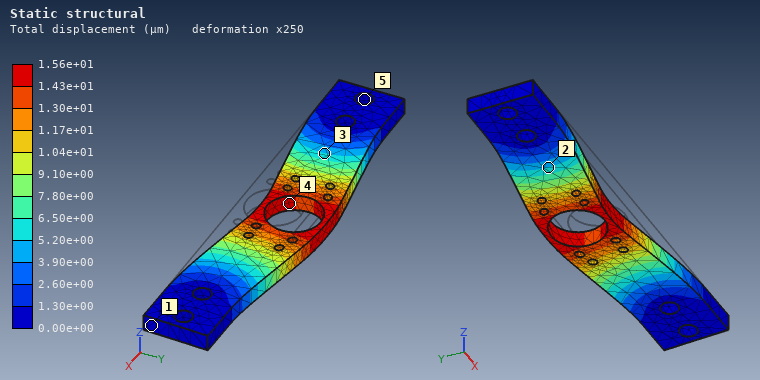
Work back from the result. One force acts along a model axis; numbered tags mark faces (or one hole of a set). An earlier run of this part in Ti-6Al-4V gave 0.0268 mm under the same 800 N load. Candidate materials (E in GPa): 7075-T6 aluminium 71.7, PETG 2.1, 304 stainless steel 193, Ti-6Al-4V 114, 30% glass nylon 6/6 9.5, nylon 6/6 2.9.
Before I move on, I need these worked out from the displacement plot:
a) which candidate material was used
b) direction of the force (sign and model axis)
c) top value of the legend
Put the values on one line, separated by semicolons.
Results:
304 stainless steel; +Y; 1.56e+01 µm
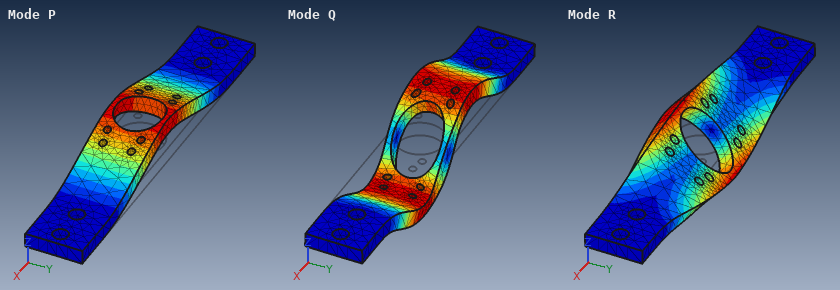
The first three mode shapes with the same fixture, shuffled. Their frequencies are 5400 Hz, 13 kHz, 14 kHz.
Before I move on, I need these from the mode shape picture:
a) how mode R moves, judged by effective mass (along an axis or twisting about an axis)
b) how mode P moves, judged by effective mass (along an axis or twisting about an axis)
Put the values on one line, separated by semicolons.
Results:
twisting about X; along Z
